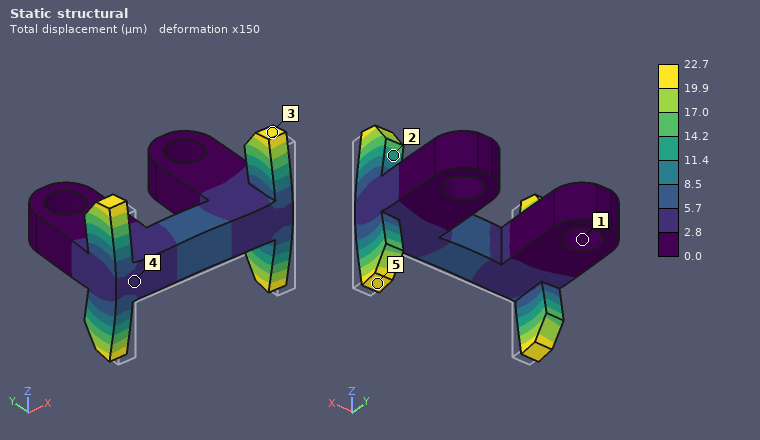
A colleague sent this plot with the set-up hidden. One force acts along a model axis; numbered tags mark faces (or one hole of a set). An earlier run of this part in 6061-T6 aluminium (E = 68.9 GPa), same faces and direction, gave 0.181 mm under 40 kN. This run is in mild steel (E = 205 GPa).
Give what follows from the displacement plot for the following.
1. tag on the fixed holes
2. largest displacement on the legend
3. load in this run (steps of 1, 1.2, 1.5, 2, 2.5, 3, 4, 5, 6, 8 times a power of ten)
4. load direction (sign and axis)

1
22.7 µm
15 kN
+Y
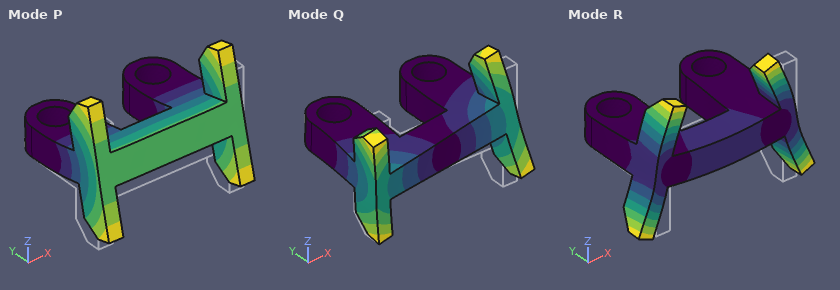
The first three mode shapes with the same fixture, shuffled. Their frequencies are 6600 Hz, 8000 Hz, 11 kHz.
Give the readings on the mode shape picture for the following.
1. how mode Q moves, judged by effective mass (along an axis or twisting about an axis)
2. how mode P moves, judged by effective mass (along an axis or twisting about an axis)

twisting about Y
along Z
